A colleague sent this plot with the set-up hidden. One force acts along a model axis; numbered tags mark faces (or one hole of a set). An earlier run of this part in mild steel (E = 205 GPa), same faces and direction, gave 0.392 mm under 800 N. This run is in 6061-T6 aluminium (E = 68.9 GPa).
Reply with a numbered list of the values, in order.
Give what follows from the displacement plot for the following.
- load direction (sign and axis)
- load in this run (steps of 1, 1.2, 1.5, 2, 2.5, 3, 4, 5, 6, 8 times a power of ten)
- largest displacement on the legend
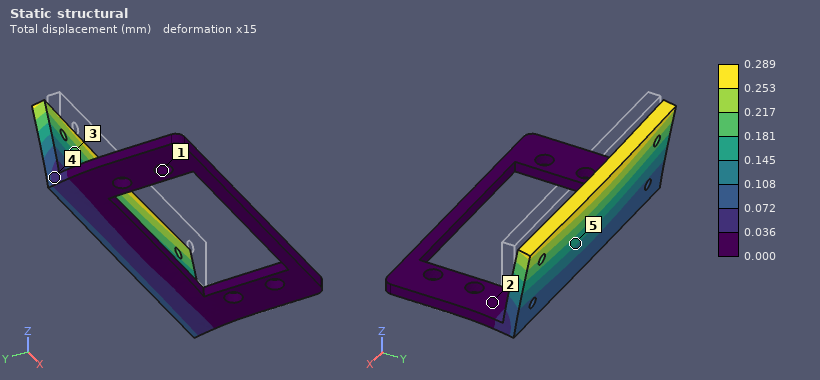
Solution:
1. +Y
2. 200 N
3. 0.289 mm
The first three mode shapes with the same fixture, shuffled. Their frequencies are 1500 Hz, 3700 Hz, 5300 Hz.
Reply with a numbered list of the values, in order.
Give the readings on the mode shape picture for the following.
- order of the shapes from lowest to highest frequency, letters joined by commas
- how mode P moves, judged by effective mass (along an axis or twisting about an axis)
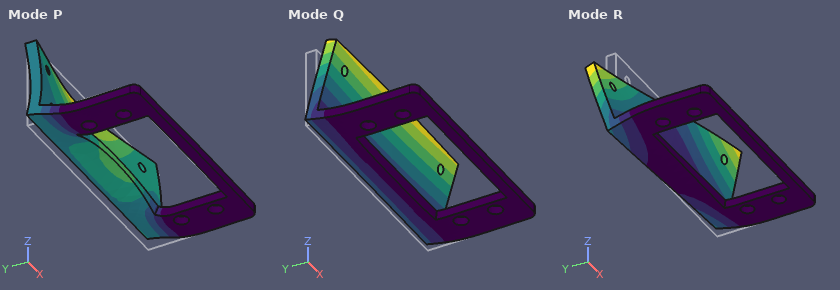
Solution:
1. Q, R, P
2. along Z
